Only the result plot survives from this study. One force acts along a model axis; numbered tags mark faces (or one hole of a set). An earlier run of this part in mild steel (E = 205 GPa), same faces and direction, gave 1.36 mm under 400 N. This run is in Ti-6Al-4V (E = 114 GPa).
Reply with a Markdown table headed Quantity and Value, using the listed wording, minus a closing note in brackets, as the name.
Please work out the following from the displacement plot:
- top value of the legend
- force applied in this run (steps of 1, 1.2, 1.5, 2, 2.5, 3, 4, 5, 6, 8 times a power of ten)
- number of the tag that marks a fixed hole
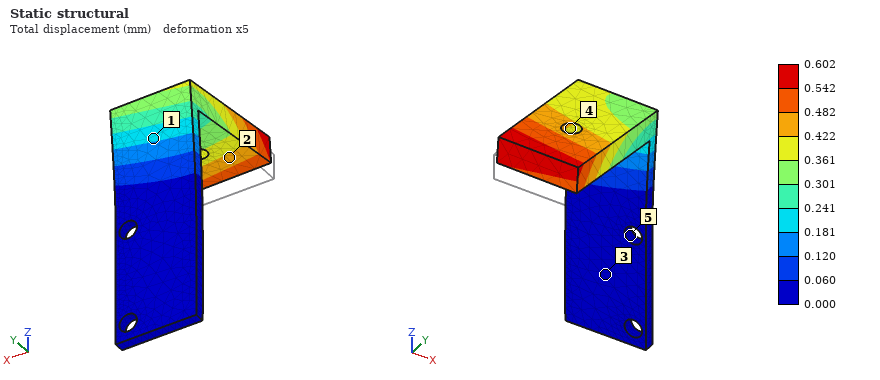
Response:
| Quantity | Value |
|---|---|
| top value of the legend | 0.602 mm |
| force applied in this run | 100 N |
| number of the tag that marks a fixed hole | 5 |
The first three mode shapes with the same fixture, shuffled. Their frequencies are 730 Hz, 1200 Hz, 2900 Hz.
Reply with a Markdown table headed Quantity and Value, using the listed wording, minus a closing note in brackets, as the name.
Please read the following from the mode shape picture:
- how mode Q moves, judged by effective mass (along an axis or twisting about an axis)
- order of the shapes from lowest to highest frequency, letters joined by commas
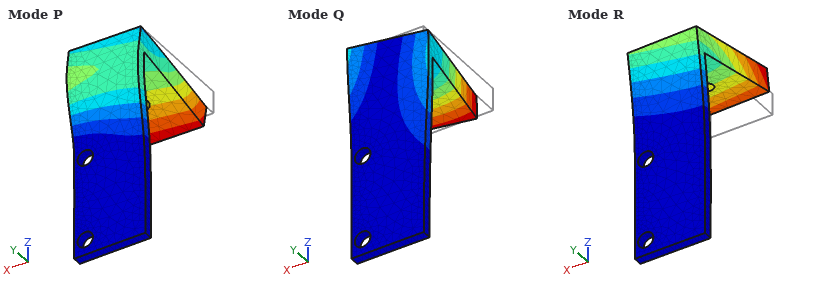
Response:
| Quantity | Value |
|---|---|
| how mode Q moves, judged by effective mass | along X |
| order of the shapes from lowest to highest frequency, letters joined by commas | R, Q, P |
